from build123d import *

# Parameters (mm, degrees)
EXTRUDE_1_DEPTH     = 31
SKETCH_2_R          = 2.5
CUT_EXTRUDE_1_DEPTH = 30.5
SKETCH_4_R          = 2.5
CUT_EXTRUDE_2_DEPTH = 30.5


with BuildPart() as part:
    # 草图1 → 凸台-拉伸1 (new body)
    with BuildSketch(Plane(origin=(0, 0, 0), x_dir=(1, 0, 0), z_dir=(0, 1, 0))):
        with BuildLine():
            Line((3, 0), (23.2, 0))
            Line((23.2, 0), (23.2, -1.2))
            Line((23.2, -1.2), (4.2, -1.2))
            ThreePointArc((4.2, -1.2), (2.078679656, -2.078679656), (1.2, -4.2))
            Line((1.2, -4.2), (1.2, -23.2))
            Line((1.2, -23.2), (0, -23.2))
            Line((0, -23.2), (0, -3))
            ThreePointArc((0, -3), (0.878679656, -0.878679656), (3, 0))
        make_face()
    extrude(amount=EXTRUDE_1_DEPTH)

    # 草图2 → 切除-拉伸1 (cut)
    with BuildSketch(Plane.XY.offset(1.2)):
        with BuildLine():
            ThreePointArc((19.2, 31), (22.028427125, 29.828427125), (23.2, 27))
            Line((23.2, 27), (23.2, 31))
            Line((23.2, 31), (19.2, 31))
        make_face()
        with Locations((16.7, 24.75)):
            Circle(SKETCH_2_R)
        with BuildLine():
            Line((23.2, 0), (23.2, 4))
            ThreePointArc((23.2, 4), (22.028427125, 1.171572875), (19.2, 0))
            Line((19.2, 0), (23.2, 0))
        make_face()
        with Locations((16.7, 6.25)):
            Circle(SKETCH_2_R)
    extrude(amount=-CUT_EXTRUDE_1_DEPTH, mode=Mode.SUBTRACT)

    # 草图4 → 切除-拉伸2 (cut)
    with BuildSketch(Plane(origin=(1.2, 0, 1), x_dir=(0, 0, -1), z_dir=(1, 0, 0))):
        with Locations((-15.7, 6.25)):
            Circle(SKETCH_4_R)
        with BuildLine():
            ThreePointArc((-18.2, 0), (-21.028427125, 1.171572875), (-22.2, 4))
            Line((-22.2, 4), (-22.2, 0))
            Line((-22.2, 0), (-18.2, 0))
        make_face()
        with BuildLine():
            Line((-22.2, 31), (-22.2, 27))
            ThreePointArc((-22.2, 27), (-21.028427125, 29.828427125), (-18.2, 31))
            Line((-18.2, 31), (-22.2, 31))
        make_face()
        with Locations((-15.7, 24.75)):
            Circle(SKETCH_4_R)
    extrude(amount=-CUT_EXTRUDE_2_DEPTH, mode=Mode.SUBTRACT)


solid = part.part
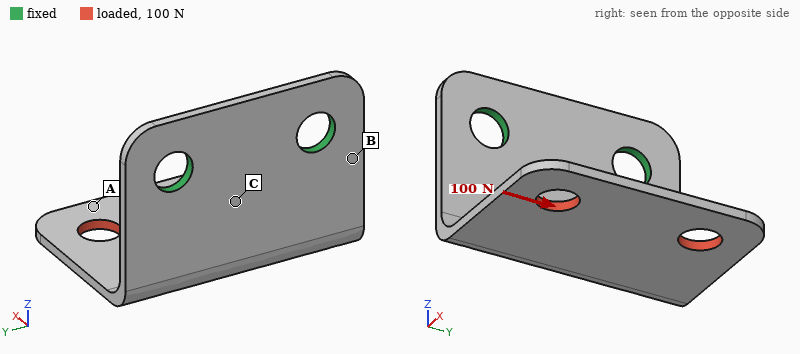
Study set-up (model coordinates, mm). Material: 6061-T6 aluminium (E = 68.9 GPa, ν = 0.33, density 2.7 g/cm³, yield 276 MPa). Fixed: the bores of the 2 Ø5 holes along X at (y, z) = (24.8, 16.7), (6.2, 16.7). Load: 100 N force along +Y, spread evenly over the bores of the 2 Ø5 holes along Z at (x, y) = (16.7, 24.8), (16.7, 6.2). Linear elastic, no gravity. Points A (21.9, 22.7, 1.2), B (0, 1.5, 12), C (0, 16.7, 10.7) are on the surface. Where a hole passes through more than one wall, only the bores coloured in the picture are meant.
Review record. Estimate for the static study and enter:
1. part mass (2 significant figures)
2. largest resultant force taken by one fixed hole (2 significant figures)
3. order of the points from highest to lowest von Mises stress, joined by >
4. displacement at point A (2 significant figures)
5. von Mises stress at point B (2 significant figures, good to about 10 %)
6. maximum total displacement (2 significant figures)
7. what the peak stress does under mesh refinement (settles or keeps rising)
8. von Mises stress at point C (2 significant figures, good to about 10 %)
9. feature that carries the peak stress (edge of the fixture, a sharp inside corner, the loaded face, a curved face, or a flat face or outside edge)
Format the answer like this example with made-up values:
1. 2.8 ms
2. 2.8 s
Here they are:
1. 4.2 g
2. 110 N
3. B > C > A
4. 0.37 mm
5. 110 MPa
6. 0.44 mm
7. keeps rising
8. 52 MPa
9. edge of the fixture
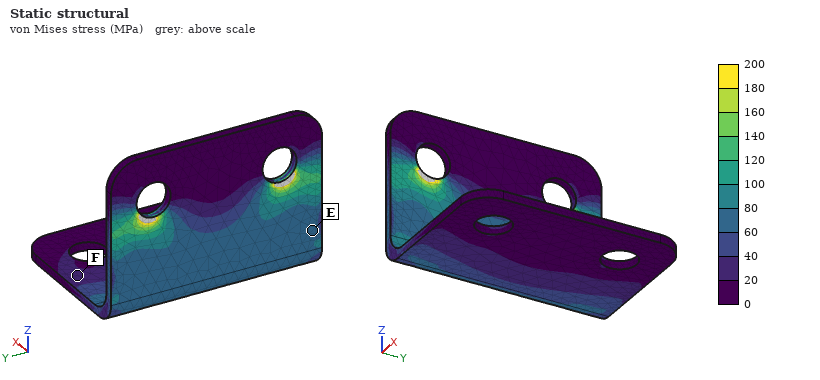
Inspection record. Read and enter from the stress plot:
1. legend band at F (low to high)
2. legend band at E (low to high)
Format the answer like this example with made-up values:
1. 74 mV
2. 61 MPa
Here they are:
1. 20 to 40 MPa
2. 60 to 80 MPa
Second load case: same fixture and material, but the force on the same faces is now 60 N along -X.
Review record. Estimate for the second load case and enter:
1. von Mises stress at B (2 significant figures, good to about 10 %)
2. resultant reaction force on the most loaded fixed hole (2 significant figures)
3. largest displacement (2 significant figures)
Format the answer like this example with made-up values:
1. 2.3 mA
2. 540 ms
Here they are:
1. 86 MPa
2. 30 N
3. 0.47 mm
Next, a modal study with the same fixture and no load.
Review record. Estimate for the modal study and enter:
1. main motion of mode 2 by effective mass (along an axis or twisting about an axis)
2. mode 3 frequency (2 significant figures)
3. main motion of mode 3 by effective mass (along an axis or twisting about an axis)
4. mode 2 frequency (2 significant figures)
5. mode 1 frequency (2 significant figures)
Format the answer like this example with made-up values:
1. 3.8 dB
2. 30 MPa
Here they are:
1. along Y
2. 3300 Hz
3. along X
4. 2100 Hz
5. 1100 Hz
